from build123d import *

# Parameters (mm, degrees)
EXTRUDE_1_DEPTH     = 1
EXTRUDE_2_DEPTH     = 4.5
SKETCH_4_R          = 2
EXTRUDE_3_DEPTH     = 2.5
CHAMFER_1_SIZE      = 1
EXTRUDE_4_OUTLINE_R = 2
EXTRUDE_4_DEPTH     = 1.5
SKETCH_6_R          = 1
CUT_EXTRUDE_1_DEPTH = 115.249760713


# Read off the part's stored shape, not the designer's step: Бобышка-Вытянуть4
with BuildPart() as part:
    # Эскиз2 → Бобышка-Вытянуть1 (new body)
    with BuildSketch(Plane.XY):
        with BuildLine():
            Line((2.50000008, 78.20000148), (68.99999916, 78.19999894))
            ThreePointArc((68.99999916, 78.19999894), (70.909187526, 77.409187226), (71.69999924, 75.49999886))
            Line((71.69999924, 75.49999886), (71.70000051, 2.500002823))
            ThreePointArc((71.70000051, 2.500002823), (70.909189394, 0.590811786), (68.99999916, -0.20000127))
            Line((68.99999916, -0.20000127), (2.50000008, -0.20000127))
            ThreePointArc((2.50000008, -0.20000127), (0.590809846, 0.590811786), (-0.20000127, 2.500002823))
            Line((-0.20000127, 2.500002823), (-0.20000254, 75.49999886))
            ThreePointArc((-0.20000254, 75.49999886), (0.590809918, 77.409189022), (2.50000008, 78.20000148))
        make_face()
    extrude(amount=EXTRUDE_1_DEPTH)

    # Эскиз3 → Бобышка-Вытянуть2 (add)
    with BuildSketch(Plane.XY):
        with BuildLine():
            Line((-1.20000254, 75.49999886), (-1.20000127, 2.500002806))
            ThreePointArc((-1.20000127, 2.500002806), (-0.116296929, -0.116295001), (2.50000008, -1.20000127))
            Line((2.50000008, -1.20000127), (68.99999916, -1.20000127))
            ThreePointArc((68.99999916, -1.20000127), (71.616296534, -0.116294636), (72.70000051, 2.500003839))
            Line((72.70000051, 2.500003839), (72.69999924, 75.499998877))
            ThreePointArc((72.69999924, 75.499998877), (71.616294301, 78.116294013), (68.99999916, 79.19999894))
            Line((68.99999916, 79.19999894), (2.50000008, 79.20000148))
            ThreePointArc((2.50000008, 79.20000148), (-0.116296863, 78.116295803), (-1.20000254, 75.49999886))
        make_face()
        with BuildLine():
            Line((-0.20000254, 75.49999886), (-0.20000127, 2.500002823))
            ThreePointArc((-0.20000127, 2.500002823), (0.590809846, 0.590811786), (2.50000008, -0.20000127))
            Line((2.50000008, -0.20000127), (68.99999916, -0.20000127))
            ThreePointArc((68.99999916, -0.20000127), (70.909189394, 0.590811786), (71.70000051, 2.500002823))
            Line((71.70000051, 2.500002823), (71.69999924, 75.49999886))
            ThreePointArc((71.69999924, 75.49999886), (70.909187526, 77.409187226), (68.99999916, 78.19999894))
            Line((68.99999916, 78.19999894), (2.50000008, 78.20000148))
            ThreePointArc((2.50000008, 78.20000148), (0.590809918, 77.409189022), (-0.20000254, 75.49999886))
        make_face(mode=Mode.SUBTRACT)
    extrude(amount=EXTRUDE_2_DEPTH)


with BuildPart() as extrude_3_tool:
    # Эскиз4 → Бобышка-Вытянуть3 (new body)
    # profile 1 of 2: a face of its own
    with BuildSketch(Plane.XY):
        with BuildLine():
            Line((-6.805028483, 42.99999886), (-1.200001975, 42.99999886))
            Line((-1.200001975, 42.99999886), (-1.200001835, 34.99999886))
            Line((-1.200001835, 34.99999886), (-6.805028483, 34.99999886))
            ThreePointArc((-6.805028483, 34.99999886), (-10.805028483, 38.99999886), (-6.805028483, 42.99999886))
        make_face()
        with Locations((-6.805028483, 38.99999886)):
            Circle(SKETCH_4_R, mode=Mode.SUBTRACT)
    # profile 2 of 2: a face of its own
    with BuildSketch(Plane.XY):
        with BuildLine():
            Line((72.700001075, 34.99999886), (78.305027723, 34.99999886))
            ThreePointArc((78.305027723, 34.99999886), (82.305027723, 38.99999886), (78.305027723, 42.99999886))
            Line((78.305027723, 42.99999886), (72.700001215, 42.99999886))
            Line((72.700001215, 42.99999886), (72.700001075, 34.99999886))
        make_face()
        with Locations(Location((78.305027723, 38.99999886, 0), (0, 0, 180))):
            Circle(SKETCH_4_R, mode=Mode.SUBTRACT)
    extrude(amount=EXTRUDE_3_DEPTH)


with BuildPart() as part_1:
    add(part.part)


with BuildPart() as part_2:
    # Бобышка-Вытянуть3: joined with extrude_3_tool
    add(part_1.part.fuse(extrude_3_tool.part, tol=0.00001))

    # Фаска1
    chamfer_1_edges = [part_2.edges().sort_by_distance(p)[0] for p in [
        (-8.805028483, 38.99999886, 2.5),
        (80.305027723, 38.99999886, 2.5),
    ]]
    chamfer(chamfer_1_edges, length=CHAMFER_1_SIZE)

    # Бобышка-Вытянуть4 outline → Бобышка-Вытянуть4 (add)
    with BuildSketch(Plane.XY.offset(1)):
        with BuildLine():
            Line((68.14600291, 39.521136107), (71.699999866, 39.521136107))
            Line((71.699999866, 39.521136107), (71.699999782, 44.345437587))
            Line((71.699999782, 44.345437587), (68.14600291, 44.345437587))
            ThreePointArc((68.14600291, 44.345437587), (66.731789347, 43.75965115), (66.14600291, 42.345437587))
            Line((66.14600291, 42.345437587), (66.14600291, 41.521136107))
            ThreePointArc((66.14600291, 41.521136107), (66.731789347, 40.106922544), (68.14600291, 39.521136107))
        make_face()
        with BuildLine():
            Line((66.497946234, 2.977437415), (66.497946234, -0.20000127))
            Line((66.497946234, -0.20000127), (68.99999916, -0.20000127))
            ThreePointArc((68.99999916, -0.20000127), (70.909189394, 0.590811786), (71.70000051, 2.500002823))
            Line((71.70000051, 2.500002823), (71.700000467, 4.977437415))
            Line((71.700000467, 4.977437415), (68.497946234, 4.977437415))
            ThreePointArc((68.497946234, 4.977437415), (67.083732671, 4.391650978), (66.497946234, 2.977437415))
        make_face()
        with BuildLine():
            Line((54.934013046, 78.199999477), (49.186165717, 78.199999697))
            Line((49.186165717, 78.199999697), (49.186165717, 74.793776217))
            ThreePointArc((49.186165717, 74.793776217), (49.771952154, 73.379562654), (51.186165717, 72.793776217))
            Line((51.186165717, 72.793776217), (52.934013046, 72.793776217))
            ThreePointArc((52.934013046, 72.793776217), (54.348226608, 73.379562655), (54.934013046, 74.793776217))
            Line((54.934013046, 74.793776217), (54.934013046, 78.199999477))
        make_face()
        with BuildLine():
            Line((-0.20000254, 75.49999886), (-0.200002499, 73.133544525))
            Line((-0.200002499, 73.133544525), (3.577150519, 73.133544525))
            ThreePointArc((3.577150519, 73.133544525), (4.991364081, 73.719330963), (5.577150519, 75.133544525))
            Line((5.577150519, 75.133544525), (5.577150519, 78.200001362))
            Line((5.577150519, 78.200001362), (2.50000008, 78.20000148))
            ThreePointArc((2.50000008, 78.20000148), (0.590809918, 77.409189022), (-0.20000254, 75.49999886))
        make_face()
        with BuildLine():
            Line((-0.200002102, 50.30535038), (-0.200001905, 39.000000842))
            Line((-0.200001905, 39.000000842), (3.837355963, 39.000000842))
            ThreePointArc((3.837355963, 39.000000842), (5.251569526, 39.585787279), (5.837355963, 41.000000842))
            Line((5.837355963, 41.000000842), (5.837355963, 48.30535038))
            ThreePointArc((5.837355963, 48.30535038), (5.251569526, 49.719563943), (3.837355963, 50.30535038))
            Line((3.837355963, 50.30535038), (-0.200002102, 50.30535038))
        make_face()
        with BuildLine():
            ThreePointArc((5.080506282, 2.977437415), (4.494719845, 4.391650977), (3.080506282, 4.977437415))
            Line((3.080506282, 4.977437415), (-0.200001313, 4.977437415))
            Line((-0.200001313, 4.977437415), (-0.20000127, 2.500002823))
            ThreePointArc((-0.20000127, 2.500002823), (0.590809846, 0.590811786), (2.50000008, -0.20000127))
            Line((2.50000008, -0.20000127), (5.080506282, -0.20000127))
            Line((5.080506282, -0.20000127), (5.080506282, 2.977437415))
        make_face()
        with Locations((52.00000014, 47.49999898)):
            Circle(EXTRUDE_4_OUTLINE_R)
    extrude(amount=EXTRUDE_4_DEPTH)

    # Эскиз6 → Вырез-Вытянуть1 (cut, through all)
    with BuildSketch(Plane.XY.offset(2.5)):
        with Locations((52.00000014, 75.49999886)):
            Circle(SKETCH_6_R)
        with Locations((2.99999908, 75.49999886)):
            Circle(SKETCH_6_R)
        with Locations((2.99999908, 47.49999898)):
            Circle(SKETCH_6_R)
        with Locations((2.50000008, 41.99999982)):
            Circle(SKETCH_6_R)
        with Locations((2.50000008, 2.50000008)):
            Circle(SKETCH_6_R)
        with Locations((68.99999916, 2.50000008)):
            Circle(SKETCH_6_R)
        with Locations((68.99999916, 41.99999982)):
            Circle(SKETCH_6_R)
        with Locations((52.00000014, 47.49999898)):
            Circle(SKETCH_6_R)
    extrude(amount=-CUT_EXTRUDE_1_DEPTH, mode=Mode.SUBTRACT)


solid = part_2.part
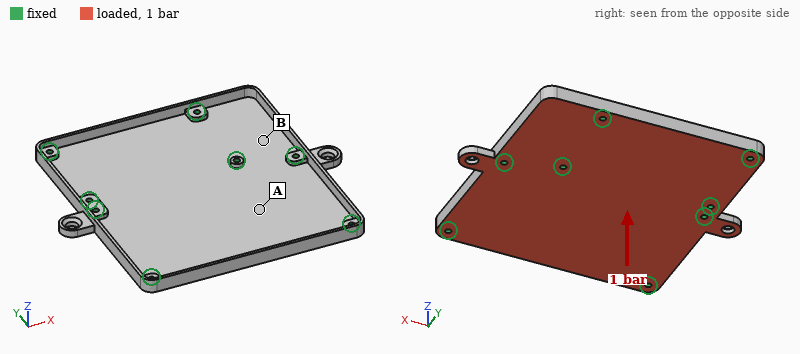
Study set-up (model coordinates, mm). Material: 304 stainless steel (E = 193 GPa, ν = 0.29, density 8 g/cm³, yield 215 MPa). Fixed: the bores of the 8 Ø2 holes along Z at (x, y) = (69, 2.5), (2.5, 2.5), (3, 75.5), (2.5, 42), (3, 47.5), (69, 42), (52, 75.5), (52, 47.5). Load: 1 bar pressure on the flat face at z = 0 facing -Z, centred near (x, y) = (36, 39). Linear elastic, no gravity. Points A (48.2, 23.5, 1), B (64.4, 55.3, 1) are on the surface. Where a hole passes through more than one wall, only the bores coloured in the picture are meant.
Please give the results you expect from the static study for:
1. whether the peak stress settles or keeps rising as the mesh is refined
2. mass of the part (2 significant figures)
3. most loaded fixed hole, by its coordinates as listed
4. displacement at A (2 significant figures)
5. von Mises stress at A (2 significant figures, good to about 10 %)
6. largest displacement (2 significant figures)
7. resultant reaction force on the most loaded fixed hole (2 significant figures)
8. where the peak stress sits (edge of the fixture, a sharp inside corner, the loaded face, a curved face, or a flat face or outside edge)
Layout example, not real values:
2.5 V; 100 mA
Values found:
keeps rising; 60 g; (52, 47.5); 0.12 mm; 52 MPa; 0.17 mm; 140 N; edge of the fixture
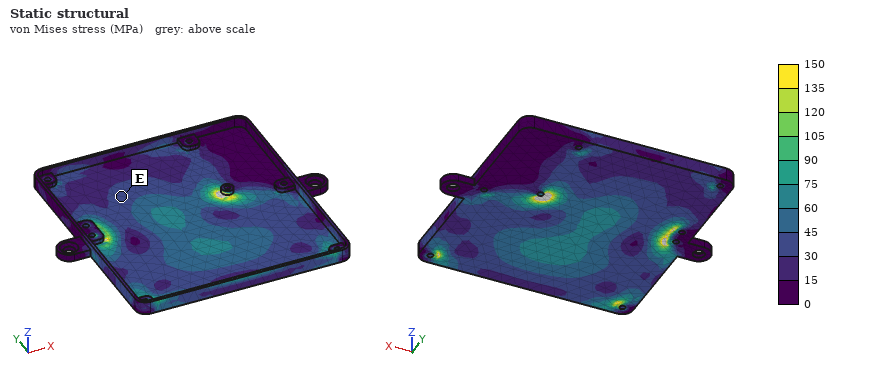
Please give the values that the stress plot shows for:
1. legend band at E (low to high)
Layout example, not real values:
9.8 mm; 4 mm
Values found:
30 to 45 MPa
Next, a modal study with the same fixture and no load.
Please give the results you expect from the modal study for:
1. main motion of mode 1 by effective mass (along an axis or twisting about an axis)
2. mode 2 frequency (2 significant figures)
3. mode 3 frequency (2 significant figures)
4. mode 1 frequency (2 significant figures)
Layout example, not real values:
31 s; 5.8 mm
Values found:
along Z; 2700 Hz; 3500 Hz; 1700 Hz
